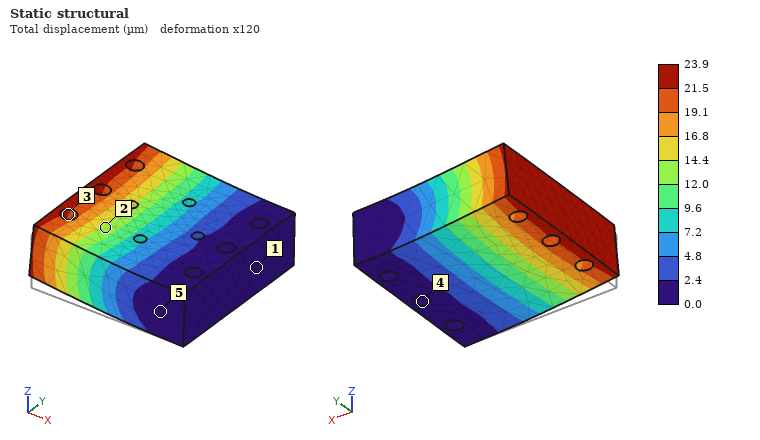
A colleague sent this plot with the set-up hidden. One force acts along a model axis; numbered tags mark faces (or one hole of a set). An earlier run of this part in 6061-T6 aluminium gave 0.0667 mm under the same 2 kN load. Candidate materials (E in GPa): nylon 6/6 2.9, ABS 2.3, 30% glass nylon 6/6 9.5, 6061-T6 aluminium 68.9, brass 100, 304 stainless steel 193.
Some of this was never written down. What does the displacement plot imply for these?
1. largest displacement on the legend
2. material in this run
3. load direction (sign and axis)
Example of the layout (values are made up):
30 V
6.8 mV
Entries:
23.9 µm
304 stainless steel
+Z
